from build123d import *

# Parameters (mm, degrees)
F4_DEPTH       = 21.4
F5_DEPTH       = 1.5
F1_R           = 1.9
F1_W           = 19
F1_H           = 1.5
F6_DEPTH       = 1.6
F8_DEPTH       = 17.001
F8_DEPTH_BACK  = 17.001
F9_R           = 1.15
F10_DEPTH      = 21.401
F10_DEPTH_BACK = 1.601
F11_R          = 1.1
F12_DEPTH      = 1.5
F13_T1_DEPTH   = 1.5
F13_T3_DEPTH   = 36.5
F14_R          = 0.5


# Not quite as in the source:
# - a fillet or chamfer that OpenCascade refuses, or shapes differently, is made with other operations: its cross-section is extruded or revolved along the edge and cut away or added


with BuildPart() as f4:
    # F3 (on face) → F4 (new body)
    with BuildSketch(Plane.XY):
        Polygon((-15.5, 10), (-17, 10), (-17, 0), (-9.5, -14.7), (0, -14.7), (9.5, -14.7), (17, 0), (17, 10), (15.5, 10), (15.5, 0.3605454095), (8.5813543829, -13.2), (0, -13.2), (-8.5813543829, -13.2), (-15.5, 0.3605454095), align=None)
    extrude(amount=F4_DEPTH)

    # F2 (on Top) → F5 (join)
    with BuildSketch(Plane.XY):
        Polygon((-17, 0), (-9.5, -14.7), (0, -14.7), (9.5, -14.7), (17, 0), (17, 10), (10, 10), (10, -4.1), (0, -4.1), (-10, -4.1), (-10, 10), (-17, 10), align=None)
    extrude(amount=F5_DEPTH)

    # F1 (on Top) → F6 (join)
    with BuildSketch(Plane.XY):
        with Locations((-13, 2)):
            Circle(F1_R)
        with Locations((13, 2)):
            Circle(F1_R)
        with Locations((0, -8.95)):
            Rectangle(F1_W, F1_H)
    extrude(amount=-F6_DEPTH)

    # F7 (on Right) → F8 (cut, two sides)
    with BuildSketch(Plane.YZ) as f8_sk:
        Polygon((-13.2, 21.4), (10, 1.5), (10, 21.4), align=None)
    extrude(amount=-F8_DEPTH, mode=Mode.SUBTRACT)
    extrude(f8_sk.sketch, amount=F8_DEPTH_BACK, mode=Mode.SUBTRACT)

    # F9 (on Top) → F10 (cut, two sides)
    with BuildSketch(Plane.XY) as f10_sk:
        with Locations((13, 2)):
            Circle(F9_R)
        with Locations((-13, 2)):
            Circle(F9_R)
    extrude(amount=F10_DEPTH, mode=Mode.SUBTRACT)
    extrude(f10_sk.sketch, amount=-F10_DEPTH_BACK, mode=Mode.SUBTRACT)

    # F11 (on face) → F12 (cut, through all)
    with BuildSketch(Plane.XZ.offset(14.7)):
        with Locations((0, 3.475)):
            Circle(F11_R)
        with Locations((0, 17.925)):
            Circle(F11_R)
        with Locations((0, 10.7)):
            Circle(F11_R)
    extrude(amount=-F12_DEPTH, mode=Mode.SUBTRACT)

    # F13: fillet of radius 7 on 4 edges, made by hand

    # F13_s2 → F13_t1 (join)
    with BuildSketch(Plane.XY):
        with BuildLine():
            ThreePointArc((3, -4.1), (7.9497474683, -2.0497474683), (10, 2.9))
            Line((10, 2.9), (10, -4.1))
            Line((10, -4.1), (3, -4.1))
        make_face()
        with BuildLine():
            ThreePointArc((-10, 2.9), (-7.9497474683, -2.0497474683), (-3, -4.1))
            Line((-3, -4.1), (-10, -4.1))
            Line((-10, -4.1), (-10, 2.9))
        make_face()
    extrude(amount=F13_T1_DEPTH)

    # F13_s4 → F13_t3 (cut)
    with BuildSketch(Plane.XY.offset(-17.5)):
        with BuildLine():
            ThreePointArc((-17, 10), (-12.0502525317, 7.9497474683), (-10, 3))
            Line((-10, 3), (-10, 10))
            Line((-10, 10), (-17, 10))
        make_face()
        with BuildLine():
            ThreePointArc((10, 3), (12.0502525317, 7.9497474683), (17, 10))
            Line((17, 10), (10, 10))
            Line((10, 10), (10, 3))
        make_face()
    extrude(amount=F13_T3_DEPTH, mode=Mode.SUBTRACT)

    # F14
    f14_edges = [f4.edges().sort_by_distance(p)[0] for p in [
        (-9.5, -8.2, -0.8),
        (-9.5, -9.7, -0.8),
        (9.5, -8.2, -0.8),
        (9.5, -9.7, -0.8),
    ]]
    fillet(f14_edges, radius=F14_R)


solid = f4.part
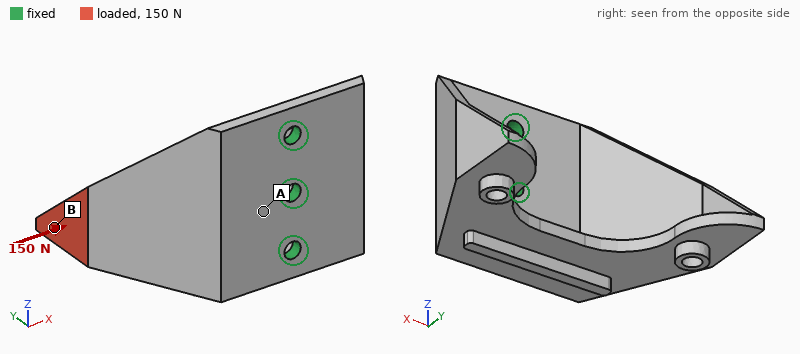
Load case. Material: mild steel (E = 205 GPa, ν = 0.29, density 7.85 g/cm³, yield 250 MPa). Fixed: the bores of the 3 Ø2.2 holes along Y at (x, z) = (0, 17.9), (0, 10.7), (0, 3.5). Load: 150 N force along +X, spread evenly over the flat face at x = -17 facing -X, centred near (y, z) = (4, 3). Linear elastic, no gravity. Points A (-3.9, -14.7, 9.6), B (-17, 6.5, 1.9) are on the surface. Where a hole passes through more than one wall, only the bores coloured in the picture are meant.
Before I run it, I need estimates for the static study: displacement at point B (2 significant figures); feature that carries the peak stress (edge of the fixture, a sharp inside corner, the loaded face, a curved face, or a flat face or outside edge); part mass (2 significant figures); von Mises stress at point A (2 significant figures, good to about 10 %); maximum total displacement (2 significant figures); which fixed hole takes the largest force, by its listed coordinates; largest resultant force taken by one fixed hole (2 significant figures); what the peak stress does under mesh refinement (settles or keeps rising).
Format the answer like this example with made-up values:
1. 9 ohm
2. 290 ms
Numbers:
1. 0.12 mm
2. edge of the fixture
3. 16 g
4. 77 MPa
5. 0.13 mm
6. (0, 3.5)
7. 140 N
8. keeps rising
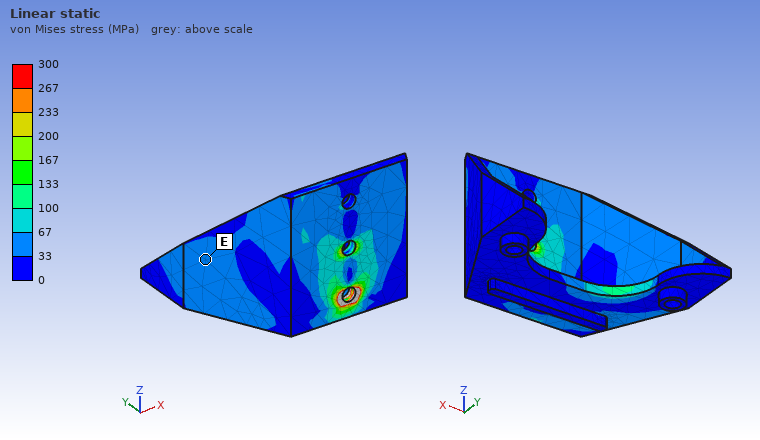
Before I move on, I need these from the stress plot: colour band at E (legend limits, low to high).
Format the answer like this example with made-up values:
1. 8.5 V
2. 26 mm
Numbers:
1. 33 to 67 MPa
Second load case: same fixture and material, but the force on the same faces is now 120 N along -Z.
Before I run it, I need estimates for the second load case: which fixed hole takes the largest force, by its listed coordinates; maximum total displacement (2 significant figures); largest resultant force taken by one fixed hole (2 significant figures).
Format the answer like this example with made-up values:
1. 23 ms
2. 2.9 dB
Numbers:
1. (0, 3.5)
2. 73 µm
3. 200 N
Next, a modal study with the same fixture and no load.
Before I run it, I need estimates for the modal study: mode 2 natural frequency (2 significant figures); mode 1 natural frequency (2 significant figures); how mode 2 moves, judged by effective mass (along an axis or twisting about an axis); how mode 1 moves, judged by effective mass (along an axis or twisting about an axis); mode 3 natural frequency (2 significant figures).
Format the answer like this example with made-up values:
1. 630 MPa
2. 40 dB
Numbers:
1. 4800 Hz
2. 2600 Hz
3. along Z
4. along X
5. 5400 Hz
